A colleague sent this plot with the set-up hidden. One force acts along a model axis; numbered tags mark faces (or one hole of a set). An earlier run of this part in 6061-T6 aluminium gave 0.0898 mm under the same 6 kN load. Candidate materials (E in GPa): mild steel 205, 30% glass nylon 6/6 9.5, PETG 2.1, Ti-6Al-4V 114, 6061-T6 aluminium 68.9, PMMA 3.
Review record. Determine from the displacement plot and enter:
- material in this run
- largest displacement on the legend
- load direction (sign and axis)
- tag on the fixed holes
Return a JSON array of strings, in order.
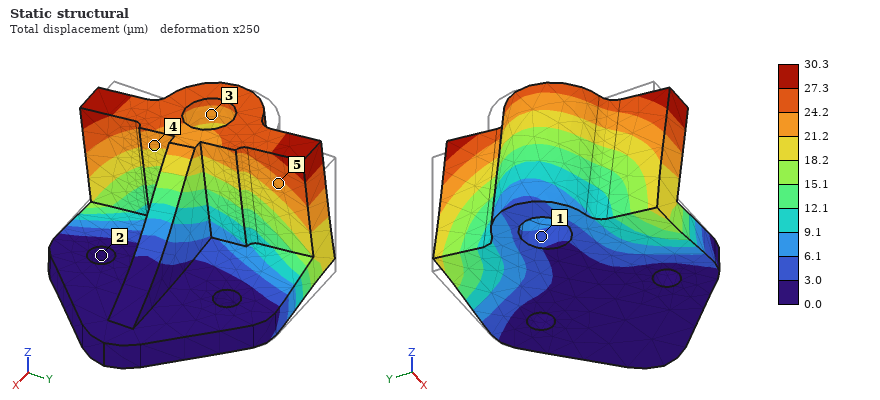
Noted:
["mild steel", "30.3 µm", "-Y", "2"]
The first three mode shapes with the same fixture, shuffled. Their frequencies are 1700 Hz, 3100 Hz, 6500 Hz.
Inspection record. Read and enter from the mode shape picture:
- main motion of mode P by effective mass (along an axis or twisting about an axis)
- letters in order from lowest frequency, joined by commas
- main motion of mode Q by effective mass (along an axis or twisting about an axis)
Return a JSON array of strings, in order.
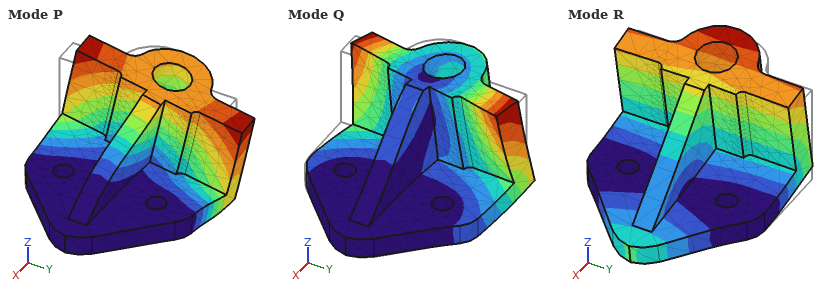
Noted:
["along Y", "R, P, Q", "along Y"]
